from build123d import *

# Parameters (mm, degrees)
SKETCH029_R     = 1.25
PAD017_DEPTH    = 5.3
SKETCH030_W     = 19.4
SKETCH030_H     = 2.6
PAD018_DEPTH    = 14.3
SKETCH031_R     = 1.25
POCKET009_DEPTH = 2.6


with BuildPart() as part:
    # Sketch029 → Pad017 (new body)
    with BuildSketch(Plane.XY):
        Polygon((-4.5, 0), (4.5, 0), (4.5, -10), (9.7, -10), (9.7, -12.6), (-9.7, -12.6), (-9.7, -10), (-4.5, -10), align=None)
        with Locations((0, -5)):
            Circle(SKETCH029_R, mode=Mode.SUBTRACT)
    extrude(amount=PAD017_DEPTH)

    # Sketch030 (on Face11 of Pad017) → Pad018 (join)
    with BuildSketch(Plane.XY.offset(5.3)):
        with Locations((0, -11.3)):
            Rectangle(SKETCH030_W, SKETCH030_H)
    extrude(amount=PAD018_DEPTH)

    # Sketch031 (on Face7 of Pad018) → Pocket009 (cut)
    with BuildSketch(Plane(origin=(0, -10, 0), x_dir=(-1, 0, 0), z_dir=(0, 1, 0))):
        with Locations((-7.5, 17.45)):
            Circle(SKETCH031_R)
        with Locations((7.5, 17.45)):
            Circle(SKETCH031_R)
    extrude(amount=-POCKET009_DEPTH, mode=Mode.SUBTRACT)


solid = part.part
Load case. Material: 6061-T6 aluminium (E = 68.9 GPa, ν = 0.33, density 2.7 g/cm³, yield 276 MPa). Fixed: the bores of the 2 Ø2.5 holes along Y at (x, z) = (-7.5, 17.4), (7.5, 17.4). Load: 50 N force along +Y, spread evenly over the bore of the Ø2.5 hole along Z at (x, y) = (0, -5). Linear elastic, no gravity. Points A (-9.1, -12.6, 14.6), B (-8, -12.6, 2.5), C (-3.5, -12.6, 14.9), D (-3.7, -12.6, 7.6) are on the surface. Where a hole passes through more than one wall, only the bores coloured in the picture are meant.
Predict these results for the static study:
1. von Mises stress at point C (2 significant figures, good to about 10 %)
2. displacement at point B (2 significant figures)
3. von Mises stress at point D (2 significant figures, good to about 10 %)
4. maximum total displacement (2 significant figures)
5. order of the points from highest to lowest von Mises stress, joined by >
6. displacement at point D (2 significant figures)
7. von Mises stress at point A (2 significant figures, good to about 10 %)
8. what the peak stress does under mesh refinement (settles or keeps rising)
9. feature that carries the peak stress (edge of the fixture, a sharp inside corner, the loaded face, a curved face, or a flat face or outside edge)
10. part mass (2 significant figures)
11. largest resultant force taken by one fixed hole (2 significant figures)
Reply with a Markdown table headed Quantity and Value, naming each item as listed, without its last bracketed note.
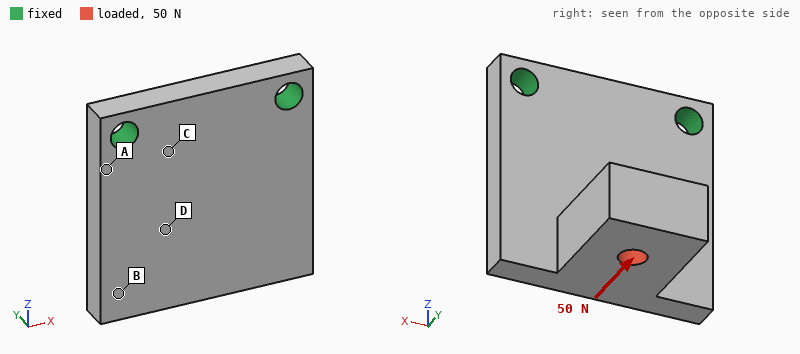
| Quantity | Value |
|---|---|
| von Mises stress at point C | 20 MPa |
| displacement at point B | 30 µm |
| von Mises stress at point D | 12 MPa |
| maximum total displacement | 51 µm |
| order of the points from highest to lowest von Mises stress, joined by > | A > C > D > B |
| displacement at point D | 17 µm |
| von Mises stress at point A | 34 MPa |
| what the peak stress does under mesh refinement | keeps rising |
| feature that carries the peak stress | edge of the fixture |
| part mass | 3.8 g |
| largest resultant force taken by one fixed hole | 25 N |
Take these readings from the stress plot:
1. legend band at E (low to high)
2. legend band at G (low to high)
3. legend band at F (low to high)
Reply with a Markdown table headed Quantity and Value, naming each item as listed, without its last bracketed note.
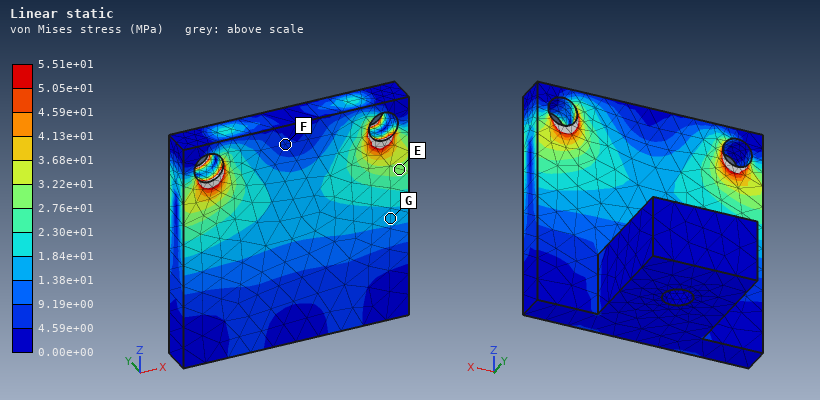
| Quantity | Value |
|---|---|
| legend band at E | 2.76e+01 to 3.22e+01 MPa |
| legend band at G | 1.38e+01 to 1.84e+01 MPa |
| legend band at F | 4.59e+00 to 9.19e+00 MPa |
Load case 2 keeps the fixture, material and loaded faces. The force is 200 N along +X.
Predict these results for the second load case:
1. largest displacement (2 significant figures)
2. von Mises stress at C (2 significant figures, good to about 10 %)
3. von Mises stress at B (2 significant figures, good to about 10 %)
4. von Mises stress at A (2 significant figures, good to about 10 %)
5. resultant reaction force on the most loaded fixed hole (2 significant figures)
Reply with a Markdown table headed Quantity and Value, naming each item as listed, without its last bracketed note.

| Quantity | Value |
|---|---|
| largest displacement | 47 µm |
| von Mises stress at C | 17 MPa |
| von Mises stress at B | 19 MPa |
| von Mises stress at A | 53 MPa |
| resultant reaction force on the most loaded fixed hole | 230 N |
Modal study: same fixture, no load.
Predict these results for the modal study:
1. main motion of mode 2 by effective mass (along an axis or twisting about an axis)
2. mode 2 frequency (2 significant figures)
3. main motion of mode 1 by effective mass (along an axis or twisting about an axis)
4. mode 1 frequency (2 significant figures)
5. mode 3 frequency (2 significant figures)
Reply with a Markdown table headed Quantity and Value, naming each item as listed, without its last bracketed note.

| Quantity | Value |
|---|---|
| main motion of mode 2 by effective mass | along X |
| mode 2 frequency | 9400 Hz |
| main motion of mode 1 by effective mass | along Y |
| mode 1 frequency | 3900 Hz |
| mode 3 frequency | 15 kHz |
